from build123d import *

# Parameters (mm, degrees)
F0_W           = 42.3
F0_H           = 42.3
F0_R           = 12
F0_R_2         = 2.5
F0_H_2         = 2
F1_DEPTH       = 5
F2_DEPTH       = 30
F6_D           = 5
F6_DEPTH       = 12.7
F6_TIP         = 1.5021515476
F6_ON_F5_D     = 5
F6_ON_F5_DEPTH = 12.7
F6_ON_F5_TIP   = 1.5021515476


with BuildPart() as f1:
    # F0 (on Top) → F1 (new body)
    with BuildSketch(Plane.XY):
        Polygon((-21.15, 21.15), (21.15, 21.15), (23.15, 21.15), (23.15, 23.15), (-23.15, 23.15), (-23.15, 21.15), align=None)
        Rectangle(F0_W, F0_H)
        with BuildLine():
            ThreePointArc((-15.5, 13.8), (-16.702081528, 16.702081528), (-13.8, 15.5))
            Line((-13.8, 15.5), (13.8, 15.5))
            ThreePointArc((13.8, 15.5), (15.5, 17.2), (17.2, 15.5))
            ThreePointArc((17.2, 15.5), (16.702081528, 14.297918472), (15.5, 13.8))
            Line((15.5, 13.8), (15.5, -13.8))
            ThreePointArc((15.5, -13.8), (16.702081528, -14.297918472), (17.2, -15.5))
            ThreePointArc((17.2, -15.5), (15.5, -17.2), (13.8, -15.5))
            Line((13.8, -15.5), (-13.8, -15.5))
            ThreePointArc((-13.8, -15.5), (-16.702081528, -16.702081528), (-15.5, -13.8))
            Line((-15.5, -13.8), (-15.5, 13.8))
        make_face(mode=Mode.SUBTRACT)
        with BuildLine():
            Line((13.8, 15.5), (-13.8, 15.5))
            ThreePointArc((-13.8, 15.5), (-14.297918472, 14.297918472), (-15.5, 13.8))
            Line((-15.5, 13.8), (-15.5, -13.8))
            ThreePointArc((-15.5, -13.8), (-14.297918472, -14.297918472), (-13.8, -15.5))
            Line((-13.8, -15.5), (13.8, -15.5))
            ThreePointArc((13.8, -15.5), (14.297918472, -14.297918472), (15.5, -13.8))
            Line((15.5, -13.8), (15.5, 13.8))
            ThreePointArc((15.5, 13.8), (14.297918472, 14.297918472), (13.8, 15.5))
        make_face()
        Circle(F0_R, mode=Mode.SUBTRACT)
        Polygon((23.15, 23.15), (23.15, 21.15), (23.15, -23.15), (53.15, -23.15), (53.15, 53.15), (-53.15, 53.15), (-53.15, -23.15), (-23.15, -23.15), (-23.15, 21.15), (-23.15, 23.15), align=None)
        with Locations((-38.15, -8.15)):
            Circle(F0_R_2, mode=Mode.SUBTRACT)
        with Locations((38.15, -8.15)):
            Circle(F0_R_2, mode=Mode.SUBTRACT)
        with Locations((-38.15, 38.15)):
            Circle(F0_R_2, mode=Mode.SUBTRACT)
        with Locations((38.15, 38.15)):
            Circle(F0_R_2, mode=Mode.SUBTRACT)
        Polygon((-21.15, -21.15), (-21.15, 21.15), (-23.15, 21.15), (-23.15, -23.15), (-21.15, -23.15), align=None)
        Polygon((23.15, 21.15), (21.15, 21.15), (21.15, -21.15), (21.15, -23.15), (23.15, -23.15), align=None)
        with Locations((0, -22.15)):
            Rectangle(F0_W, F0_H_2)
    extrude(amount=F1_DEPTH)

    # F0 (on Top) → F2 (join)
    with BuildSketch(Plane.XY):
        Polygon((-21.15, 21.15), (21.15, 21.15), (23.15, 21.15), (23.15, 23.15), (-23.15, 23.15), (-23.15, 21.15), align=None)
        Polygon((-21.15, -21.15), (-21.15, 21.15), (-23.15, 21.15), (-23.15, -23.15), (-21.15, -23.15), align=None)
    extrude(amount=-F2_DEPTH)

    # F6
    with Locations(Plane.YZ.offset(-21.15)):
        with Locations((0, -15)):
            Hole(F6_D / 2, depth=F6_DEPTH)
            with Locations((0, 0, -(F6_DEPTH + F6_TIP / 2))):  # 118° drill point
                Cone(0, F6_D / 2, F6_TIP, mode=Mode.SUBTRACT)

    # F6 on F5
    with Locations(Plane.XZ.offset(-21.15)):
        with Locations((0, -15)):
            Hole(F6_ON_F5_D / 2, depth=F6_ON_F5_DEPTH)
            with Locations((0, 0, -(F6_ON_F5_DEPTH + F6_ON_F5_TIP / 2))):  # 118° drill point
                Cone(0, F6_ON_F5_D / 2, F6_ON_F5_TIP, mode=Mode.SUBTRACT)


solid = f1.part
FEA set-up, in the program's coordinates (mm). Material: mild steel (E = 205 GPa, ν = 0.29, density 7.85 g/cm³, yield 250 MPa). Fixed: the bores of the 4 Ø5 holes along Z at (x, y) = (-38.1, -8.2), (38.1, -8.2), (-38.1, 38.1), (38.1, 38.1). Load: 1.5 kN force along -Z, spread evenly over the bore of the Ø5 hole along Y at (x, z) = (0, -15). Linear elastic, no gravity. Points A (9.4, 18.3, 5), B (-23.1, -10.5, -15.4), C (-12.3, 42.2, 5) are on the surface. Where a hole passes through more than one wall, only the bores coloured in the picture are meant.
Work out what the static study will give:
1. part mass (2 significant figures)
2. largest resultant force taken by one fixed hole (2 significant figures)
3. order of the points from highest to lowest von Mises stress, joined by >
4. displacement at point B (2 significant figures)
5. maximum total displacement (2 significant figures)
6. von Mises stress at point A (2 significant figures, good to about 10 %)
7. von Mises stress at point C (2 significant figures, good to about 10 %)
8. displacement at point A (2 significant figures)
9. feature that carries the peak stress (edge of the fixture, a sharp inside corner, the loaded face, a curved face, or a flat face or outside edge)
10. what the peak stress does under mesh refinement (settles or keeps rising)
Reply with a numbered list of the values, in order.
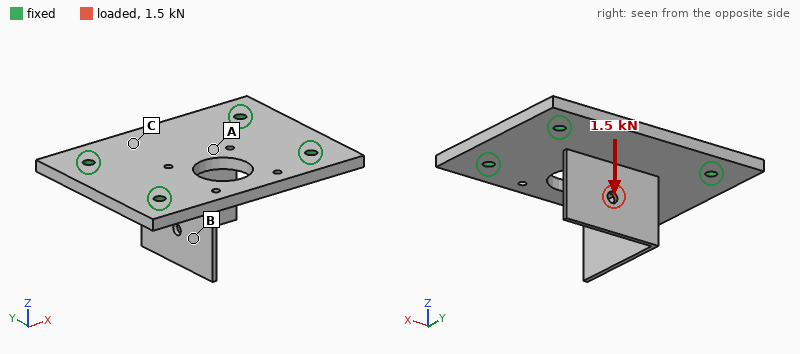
1. 340 g
2. 530 N
3. A > C > B
4. 8.4 µm
5. 21 µm
6. 20 MPa
7. 13 MPa
8. 19 µm
9. edge of the fixture
10. keeps rising
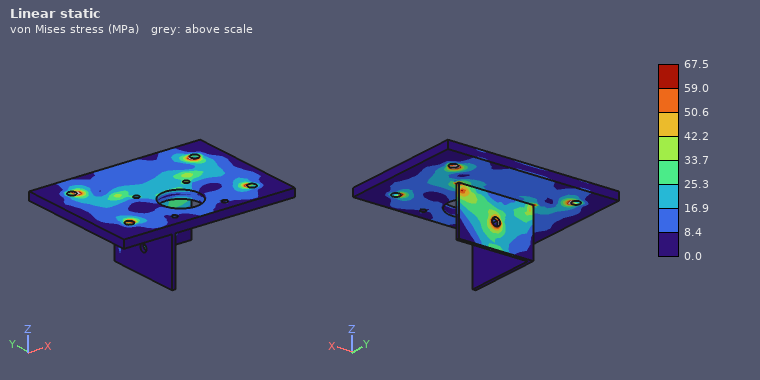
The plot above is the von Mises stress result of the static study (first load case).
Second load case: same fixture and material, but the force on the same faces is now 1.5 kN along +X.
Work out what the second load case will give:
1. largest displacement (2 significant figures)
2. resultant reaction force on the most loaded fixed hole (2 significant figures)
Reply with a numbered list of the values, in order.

1. 18 µm
2. 600 N
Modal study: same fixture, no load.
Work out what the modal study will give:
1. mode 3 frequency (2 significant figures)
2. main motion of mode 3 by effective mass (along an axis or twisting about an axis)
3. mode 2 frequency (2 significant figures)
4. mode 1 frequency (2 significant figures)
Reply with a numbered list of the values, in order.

1. 4400 Hz
2. along Z
3. 2500 Hz
4. 2300 Hz
